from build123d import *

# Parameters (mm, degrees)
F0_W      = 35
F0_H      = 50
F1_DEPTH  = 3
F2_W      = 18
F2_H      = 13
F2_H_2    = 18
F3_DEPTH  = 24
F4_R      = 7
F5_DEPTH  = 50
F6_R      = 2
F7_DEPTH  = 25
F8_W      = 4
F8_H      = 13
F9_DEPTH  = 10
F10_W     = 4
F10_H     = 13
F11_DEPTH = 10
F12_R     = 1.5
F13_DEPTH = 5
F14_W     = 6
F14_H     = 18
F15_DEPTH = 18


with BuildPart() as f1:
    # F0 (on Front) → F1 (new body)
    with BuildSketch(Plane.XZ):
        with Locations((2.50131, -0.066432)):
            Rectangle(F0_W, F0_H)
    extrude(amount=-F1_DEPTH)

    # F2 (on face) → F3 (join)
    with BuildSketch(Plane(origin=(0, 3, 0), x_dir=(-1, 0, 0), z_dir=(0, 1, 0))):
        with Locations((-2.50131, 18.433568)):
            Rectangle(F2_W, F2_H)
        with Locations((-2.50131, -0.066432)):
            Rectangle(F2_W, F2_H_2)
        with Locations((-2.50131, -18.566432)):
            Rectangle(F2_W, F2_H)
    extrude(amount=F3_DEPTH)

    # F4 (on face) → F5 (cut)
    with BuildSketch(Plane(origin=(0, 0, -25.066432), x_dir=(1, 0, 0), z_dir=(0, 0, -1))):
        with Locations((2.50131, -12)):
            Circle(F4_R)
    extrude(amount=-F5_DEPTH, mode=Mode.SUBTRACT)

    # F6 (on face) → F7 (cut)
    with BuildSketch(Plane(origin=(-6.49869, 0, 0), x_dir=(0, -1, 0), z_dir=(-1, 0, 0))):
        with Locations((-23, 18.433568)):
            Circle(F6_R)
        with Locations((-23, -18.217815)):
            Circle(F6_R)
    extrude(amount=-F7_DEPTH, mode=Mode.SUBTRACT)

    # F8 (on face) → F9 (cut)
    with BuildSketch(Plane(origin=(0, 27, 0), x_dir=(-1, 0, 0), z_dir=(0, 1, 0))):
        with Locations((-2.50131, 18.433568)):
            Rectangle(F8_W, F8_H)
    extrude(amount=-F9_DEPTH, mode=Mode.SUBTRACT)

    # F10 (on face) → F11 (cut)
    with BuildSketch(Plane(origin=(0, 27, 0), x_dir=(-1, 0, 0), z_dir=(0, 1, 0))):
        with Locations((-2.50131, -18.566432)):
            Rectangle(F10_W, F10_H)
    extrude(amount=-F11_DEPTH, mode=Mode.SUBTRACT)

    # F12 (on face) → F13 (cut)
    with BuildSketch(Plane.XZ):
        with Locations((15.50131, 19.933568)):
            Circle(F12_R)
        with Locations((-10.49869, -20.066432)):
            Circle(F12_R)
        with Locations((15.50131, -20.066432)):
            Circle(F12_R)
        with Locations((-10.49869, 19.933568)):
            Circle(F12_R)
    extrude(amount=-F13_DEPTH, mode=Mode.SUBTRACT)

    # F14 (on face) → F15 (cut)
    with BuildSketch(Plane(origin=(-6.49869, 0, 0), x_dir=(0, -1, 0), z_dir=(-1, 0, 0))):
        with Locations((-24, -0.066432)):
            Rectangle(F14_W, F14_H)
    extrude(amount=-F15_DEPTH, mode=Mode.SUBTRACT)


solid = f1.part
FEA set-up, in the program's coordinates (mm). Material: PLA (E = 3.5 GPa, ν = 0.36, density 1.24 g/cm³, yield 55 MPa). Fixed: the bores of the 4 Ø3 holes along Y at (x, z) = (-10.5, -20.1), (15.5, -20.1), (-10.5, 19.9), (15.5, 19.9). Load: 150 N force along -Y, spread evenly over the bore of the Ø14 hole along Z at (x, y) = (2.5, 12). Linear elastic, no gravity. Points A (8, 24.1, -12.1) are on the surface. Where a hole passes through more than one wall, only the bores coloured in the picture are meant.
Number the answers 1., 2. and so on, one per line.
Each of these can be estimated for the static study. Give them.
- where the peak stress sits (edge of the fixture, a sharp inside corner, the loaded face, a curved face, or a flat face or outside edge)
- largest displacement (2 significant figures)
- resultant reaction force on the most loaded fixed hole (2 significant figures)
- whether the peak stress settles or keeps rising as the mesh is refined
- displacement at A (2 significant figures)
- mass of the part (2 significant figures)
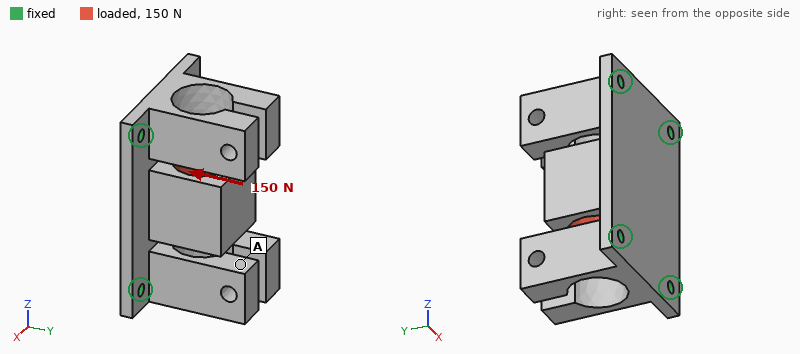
1. edge of the fixture
2. 0.15 mm
3. 43 N
4. keeps rising
5. 0.13 mm
6. 18 g
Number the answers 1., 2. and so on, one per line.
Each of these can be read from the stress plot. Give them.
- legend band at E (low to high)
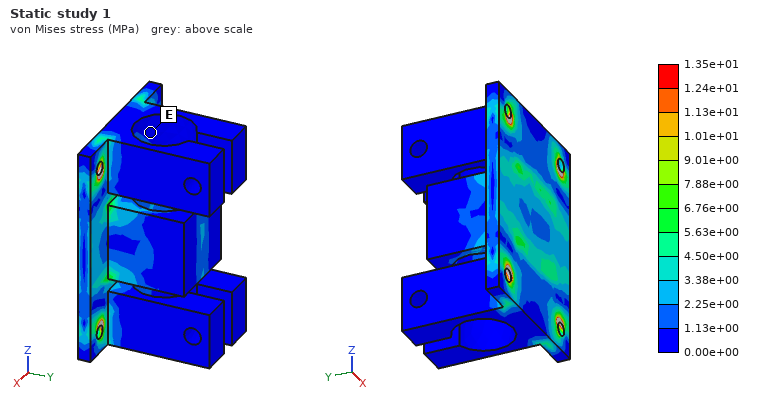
1. 0.00e+00 to 1.13e+00 MPa
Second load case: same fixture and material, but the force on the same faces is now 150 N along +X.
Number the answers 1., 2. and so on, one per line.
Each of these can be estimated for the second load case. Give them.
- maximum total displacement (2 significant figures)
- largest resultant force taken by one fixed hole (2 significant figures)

1. 0.18 mm
2. 58 N
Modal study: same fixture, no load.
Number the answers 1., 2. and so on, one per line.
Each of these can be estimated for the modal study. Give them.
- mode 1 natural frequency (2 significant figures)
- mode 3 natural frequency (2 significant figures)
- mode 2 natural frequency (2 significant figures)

1. 960 Hz
2. 980 Hz
3. 960 Hz
